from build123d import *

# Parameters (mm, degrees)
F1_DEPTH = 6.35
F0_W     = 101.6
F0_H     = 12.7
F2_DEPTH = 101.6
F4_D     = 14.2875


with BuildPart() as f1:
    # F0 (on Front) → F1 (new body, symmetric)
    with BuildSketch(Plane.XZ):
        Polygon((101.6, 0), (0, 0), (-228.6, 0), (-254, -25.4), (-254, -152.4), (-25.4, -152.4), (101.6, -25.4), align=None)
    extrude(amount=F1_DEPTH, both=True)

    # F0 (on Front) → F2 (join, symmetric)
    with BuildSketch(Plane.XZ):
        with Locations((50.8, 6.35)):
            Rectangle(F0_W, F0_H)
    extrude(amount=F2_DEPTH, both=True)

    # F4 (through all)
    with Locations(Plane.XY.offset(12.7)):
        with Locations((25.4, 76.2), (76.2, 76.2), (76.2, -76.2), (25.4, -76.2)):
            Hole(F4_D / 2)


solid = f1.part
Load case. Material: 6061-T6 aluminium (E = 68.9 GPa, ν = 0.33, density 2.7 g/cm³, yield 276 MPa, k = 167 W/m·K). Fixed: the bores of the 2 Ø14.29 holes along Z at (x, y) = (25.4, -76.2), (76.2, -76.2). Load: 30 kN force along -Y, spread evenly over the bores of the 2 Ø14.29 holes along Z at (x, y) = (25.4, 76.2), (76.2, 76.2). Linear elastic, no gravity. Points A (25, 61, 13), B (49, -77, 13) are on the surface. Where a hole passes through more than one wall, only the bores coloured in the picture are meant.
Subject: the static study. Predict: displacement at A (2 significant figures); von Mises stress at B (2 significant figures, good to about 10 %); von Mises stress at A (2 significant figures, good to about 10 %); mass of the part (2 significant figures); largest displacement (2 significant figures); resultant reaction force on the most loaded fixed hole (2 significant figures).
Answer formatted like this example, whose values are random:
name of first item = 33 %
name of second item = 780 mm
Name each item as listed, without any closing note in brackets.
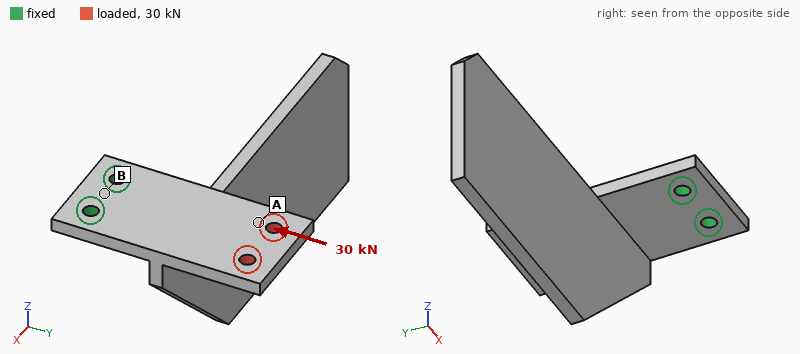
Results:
displacement at A = 52 µm
von Mises stress at B = 9.0 MPa
von Mises stress at A = 28 MPa
mass of the part = 2.3 kg
largest displacement = 65 µm
resultant reaction force on the most loaded fixed hole = 15 kN
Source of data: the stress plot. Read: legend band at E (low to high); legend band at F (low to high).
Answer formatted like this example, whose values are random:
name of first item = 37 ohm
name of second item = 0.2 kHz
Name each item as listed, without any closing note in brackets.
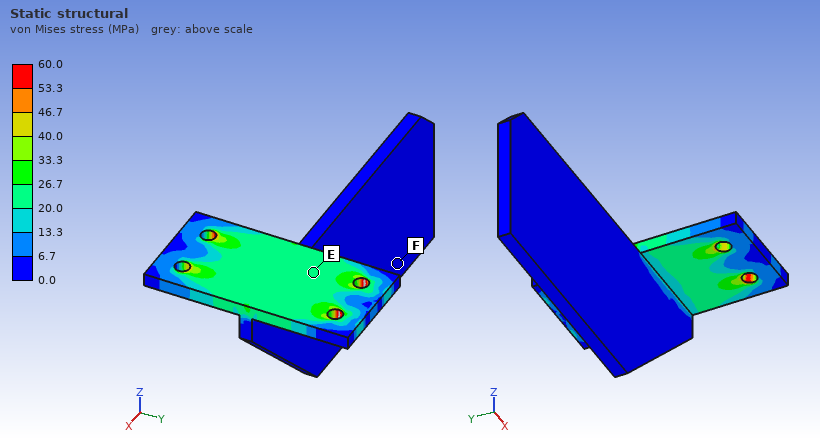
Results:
legend band at E = 20.0 to 26.7 MPa
legend band at F = 0.0 to 6.7 MPa
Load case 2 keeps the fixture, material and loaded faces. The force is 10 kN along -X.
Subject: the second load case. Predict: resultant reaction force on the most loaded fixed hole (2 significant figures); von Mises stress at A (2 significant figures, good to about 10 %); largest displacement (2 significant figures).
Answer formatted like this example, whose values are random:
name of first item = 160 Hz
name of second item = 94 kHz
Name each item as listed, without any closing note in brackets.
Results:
resultant reaction force on the most loaded fixed hole = 26 kN
von Mises stress at A = 20 MPa
largest displacement = 0.47 mm
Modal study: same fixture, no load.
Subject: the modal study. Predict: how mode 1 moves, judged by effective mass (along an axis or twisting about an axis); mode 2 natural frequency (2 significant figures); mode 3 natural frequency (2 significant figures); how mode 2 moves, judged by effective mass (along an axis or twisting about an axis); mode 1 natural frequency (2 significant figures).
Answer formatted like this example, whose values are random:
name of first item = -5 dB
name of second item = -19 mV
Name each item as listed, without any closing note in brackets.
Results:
how mode 1 moves, judged by effective mass = along Y
mode 2 natural frequency = 130 Hz
mode 3 natural frequency = 220 Hz
how mode 2 moves, judged by effective mass = along Z
mode 1 natural frequency = 87 Hz
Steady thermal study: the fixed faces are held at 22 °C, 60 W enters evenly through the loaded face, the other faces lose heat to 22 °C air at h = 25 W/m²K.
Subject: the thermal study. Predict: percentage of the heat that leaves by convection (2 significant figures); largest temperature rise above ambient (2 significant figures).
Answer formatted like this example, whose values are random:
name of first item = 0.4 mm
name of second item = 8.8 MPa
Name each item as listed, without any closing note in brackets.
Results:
percentage of the heat that leaves by convection = 48 %
largest temperature rise above ambient = 31 K
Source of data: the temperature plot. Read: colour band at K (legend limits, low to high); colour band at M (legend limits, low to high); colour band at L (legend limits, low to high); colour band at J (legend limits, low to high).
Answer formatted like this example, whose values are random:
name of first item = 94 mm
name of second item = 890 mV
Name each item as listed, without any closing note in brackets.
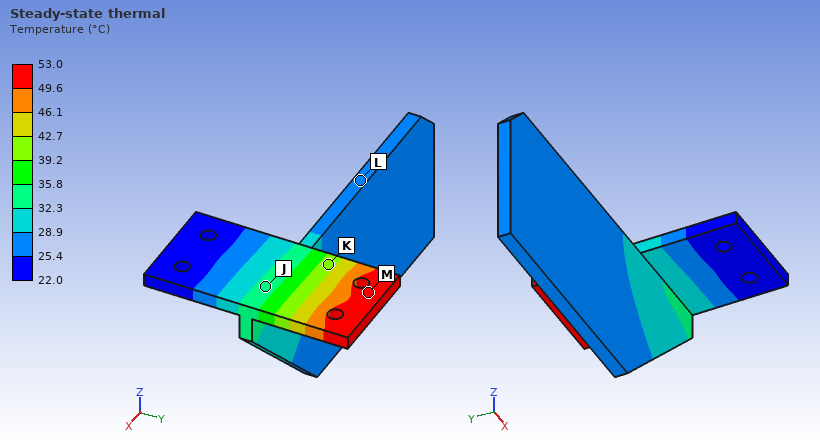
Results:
colour band at K = 39.2 to 42.7 °C
colour band at M = 49.6 to 53.0 °C
colour band at L = 25.4 to 28.9 °C
colour band at J = 32.3 to 35.8 °C
